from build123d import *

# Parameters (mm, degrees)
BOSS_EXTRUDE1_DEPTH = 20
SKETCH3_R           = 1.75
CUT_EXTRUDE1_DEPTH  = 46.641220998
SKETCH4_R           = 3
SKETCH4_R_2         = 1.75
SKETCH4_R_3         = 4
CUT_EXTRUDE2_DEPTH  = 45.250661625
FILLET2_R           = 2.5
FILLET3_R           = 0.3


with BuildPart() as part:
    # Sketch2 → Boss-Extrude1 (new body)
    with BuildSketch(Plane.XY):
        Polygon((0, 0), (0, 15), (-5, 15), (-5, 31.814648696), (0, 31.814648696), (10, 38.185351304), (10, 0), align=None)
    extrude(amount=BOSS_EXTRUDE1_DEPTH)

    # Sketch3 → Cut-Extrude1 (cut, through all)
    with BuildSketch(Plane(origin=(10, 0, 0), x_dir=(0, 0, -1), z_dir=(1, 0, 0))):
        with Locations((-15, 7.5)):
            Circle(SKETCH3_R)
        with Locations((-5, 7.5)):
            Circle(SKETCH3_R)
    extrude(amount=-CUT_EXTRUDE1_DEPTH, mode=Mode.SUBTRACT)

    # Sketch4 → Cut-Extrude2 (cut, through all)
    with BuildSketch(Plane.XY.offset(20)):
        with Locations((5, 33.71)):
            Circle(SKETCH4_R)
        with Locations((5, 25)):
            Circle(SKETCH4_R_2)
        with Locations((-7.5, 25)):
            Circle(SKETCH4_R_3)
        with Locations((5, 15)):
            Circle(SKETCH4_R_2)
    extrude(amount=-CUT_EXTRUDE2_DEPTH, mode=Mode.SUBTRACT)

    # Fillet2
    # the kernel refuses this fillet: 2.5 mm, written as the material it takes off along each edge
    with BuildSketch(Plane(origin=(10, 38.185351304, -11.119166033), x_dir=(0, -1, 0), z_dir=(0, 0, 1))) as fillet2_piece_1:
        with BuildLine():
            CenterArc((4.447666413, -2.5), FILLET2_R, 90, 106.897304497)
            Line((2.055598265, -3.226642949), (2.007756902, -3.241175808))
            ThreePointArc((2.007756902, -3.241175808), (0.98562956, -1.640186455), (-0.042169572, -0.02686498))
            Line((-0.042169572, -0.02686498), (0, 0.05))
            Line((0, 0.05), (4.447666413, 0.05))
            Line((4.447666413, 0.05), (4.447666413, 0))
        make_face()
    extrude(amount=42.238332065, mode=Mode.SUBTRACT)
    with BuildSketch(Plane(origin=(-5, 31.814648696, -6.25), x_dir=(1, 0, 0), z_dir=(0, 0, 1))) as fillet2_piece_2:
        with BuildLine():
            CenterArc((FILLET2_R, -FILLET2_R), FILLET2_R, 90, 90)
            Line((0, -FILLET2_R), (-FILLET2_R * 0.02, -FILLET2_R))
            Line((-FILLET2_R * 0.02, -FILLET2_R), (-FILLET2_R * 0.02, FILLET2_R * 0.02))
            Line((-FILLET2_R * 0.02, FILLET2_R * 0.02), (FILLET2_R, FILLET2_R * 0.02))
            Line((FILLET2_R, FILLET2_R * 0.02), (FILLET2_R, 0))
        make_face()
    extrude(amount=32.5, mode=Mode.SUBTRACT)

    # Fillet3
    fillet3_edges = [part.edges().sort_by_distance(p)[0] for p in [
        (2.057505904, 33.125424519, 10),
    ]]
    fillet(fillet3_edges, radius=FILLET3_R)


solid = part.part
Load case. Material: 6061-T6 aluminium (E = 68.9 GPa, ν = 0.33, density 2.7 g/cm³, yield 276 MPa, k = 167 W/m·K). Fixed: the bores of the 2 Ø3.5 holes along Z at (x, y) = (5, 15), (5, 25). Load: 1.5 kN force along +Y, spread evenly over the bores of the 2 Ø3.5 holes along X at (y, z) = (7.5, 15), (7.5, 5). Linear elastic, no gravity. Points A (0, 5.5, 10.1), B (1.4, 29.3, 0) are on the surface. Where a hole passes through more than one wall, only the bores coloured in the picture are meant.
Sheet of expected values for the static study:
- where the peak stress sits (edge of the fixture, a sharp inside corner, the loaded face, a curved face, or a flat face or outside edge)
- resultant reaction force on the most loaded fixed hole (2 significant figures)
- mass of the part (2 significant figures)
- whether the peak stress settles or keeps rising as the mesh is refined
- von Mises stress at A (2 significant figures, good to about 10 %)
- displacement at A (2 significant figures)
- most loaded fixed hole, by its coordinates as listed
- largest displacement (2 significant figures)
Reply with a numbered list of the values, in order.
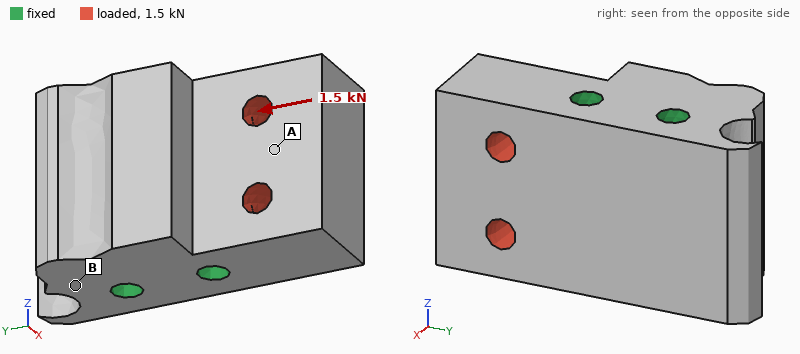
1. edge of the fixture
2. 1.3 kN
3. 20 g
4. keeps rising
5. 4.5 MPa
6. 0.76 µm
7. (5, 15)
8. 1.3 µm
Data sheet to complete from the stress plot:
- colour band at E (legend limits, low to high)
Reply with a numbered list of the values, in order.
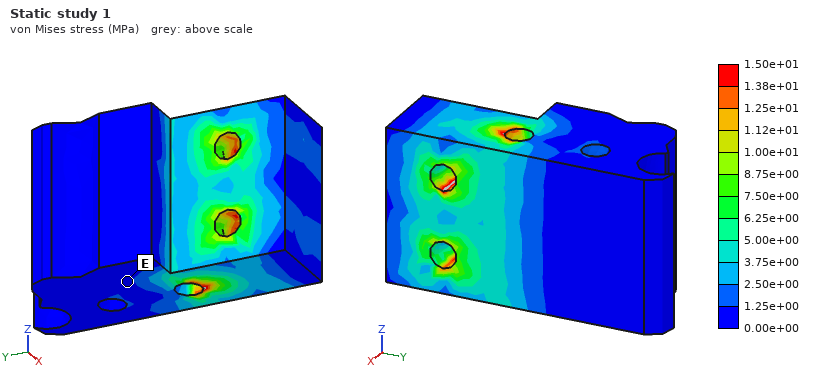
1. 0.00e+00 to 1.25e+00 MPa
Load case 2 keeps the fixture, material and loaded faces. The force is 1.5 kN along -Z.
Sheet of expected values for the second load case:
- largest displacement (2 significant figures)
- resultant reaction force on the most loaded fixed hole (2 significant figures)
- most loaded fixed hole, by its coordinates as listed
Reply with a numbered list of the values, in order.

1. 4.2 µm
2. 1.5 kN
3. (5, 15)
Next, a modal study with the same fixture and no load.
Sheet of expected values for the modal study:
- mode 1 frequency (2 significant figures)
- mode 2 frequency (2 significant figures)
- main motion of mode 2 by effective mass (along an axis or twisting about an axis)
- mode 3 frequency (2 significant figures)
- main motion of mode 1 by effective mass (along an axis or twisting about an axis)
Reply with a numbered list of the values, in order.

1. 24 kHz
2. 37 kHz
3. along Z
4. 40 kHz
5. along X
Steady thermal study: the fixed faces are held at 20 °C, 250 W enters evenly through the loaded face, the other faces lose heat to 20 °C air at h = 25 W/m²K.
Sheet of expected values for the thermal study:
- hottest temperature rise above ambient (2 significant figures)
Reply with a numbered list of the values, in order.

1. 67 K
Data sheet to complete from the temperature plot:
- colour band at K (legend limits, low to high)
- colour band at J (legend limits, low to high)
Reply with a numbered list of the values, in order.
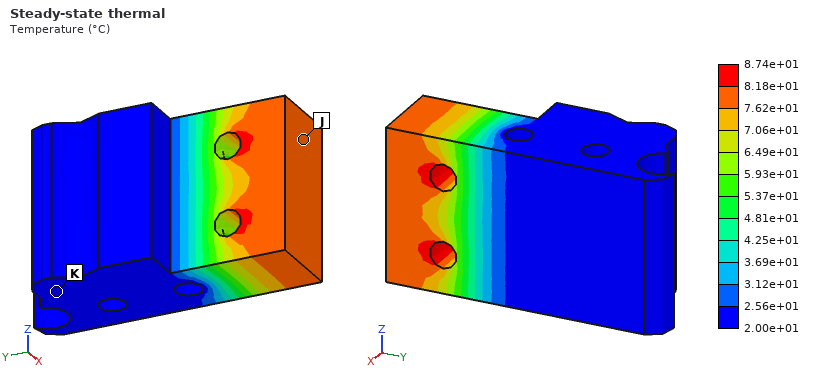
1. 2.00e+01 to 2.56e+01 °C
2. 7.62e+01 to 8.18e+01 °C
